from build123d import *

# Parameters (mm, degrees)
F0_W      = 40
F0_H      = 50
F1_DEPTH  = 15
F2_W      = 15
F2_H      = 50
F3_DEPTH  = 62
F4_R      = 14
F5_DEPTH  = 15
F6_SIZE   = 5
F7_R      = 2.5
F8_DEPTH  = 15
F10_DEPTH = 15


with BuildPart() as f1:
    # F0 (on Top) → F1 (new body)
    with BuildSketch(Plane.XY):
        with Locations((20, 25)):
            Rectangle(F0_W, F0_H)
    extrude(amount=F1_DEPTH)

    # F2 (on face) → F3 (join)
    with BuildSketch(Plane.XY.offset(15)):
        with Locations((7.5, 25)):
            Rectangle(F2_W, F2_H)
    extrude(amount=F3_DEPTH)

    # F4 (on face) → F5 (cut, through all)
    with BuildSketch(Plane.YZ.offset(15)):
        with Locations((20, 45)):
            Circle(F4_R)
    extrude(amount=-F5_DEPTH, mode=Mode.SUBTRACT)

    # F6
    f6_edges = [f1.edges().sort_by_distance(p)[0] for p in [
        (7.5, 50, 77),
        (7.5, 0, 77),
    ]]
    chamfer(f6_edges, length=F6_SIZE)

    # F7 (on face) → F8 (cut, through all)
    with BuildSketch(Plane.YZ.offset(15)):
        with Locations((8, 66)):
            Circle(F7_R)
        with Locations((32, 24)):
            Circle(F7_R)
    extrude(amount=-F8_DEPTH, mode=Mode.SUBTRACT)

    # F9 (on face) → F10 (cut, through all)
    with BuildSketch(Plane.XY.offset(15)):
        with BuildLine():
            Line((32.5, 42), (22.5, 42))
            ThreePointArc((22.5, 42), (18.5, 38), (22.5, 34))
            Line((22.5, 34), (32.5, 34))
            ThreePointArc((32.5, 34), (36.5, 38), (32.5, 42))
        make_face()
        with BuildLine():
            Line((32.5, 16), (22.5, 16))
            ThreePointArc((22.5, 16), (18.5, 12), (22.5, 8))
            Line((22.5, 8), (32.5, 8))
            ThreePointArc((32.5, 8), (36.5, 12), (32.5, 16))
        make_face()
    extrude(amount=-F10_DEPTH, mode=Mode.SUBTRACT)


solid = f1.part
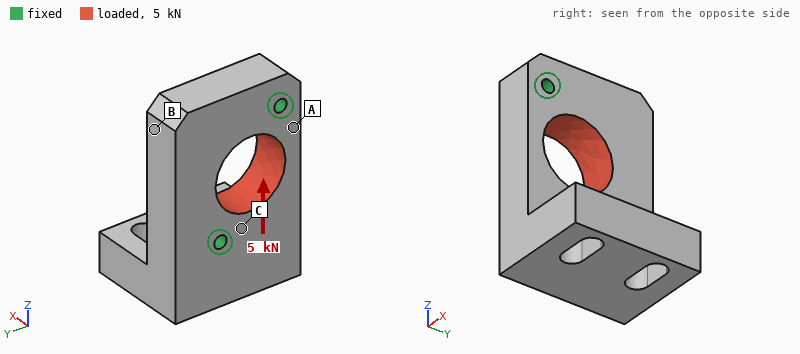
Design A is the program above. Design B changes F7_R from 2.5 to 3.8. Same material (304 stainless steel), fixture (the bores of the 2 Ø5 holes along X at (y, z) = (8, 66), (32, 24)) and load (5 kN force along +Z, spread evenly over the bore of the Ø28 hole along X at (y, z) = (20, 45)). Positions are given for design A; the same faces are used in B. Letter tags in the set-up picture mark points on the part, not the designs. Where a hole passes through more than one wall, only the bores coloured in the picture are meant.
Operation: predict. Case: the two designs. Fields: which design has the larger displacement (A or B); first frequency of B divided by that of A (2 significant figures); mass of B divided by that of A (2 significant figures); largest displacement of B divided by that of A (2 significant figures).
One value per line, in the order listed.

A
1.1
0.99
0.89
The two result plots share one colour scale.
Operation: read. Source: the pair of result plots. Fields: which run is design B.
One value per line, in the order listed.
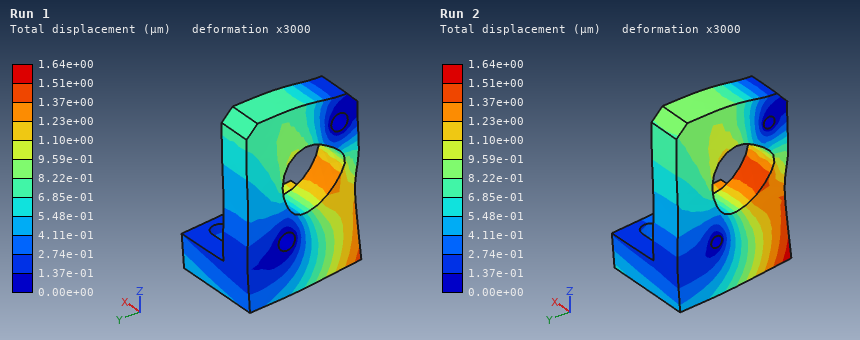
Run 1
